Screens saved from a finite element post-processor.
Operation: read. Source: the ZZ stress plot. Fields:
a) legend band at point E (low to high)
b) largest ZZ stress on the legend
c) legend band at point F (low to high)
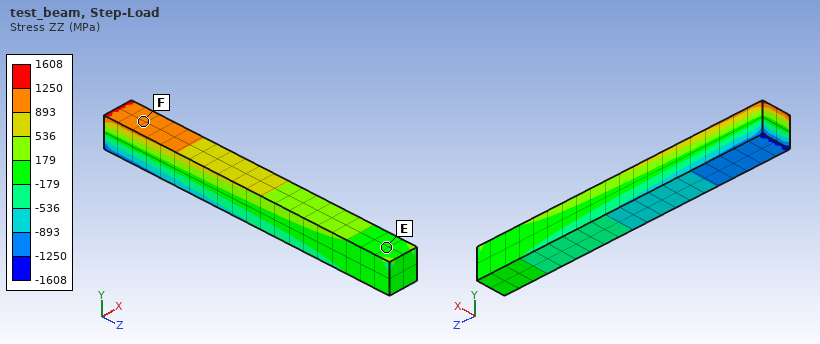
-179 to 179 MPa
1608 MPa
893 to 1250 MPa
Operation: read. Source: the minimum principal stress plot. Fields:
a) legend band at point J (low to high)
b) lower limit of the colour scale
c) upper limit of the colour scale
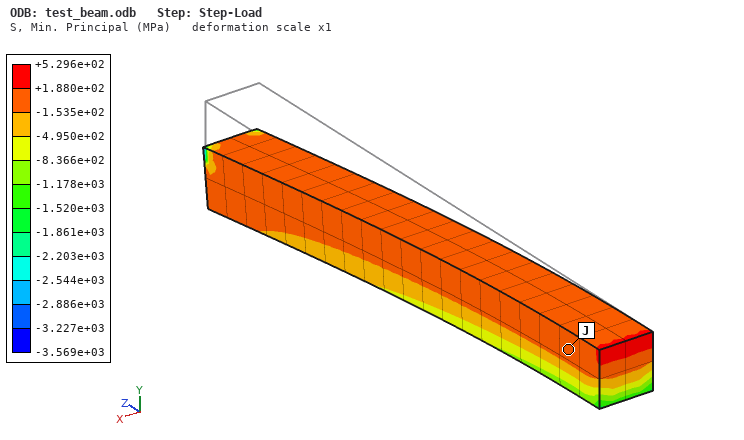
-1.535e+02 to +1.880e+02 MPa
-3.569e+03 MPa
+5.296e+02 MPa
